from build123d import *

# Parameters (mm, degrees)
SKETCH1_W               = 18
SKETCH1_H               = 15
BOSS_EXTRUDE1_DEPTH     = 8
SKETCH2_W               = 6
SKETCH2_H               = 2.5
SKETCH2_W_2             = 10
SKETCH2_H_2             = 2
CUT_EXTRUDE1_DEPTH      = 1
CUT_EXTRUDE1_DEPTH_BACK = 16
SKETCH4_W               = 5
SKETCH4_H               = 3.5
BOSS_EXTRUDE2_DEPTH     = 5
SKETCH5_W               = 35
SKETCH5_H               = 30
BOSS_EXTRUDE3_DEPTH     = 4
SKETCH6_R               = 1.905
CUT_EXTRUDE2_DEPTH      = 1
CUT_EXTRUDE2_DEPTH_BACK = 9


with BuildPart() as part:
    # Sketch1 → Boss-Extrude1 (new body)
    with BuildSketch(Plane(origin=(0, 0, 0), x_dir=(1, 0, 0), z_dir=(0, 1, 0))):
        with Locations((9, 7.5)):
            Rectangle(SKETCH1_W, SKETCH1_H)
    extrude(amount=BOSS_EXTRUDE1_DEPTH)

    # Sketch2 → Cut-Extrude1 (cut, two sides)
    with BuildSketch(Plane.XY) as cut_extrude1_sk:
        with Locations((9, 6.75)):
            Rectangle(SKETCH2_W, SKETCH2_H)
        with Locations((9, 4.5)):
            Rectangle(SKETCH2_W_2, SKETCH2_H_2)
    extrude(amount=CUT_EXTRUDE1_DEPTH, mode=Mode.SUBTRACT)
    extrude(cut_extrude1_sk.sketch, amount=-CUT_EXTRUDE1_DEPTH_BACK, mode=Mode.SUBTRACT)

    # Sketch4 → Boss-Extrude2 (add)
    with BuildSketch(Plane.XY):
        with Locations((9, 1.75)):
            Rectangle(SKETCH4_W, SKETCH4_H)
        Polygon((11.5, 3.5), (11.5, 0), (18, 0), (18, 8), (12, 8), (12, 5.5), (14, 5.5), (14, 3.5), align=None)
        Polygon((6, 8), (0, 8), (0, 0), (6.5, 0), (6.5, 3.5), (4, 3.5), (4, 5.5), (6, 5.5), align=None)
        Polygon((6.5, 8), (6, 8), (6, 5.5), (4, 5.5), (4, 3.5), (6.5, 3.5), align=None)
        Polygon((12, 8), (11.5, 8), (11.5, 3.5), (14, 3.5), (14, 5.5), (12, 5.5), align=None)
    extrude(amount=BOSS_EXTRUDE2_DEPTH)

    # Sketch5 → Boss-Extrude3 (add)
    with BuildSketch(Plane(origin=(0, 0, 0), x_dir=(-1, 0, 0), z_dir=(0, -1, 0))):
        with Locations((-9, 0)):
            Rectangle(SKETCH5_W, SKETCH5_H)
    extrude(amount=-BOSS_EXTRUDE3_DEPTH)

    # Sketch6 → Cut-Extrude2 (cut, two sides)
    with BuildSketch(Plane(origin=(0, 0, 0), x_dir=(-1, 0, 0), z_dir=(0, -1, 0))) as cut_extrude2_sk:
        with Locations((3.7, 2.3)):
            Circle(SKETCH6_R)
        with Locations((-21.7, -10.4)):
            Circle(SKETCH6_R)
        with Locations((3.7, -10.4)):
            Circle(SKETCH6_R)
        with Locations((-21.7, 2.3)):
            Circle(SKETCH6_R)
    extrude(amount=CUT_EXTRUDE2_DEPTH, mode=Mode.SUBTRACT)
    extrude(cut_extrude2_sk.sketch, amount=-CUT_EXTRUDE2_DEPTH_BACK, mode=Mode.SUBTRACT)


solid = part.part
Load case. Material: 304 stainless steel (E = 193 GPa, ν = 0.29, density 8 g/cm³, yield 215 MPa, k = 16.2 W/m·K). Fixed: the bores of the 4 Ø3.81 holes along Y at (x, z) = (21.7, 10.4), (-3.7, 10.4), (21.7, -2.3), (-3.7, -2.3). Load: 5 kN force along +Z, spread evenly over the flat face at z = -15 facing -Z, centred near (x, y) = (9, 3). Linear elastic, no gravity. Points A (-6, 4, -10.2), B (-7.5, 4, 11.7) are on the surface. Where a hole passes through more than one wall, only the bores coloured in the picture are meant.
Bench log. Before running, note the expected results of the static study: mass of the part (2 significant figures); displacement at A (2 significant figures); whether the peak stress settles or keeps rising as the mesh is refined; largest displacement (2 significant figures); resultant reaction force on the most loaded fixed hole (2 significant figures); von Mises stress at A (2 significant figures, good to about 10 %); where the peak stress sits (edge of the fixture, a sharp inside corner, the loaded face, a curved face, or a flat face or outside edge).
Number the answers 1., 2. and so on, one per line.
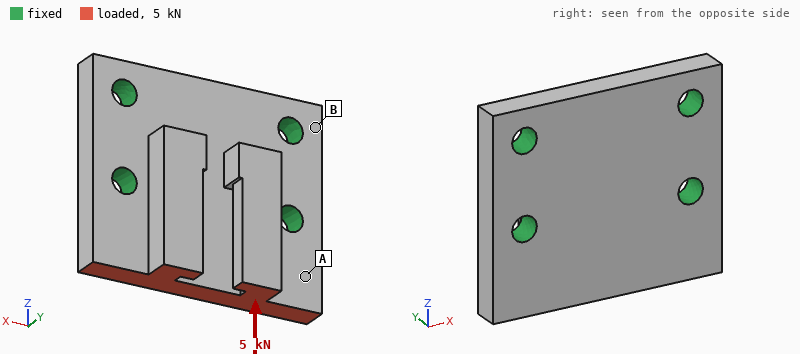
1. 39 g
2. 2.0 µm
3. keeps rising
4. 5.5 µm
5. 2.0 kN
6. 34 MPa
7. edge of the fixture
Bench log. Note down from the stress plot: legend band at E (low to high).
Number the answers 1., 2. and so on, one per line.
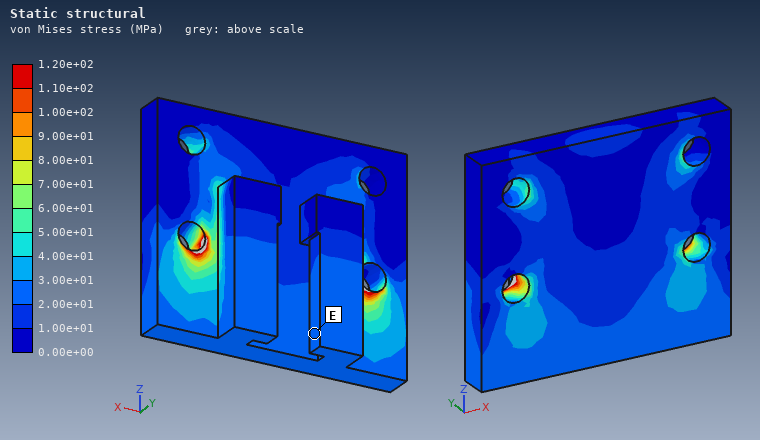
1. 2.00e+01 to 3.00e+01 MPa
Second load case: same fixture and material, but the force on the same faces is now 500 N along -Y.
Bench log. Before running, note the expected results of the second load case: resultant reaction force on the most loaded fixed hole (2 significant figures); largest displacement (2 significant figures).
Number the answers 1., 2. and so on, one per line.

1. 390 N
2. 8.2 µm
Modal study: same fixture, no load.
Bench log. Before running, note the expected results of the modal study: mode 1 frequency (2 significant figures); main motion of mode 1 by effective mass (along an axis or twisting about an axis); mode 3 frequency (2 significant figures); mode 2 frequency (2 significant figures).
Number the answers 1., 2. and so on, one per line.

1. 16 kHz
2. along Y
3. 27 kHz
4. 26 kHz
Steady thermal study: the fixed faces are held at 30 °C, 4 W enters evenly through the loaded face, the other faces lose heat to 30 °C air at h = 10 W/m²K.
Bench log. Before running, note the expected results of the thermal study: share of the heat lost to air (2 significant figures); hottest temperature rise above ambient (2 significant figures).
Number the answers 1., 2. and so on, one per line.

1. 4.7 %
2. 21 K
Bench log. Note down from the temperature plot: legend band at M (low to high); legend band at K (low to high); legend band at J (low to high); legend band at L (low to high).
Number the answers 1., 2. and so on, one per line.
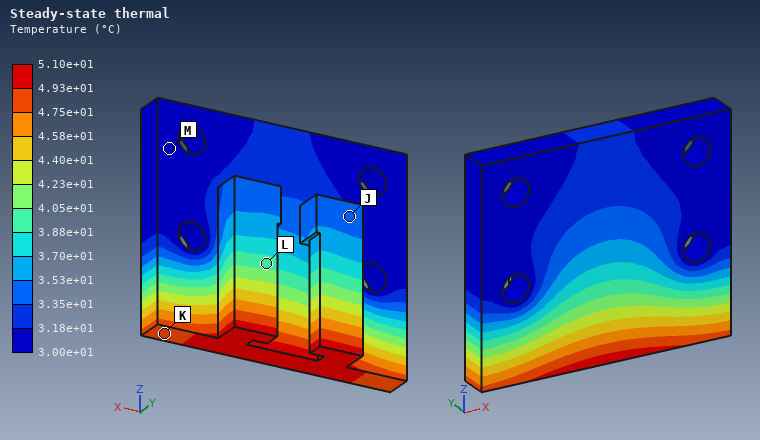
1. 3.00e+01 to 3.18e+01 °C
2. 4.75e+01 to 4.93e+01 °C
3. 3.35e+01 to 3.53e+01 °C
4. 3.88e+01 to 4.05e+01 °C
